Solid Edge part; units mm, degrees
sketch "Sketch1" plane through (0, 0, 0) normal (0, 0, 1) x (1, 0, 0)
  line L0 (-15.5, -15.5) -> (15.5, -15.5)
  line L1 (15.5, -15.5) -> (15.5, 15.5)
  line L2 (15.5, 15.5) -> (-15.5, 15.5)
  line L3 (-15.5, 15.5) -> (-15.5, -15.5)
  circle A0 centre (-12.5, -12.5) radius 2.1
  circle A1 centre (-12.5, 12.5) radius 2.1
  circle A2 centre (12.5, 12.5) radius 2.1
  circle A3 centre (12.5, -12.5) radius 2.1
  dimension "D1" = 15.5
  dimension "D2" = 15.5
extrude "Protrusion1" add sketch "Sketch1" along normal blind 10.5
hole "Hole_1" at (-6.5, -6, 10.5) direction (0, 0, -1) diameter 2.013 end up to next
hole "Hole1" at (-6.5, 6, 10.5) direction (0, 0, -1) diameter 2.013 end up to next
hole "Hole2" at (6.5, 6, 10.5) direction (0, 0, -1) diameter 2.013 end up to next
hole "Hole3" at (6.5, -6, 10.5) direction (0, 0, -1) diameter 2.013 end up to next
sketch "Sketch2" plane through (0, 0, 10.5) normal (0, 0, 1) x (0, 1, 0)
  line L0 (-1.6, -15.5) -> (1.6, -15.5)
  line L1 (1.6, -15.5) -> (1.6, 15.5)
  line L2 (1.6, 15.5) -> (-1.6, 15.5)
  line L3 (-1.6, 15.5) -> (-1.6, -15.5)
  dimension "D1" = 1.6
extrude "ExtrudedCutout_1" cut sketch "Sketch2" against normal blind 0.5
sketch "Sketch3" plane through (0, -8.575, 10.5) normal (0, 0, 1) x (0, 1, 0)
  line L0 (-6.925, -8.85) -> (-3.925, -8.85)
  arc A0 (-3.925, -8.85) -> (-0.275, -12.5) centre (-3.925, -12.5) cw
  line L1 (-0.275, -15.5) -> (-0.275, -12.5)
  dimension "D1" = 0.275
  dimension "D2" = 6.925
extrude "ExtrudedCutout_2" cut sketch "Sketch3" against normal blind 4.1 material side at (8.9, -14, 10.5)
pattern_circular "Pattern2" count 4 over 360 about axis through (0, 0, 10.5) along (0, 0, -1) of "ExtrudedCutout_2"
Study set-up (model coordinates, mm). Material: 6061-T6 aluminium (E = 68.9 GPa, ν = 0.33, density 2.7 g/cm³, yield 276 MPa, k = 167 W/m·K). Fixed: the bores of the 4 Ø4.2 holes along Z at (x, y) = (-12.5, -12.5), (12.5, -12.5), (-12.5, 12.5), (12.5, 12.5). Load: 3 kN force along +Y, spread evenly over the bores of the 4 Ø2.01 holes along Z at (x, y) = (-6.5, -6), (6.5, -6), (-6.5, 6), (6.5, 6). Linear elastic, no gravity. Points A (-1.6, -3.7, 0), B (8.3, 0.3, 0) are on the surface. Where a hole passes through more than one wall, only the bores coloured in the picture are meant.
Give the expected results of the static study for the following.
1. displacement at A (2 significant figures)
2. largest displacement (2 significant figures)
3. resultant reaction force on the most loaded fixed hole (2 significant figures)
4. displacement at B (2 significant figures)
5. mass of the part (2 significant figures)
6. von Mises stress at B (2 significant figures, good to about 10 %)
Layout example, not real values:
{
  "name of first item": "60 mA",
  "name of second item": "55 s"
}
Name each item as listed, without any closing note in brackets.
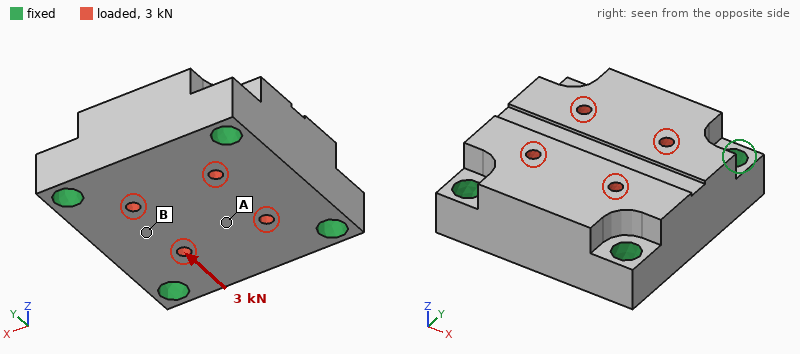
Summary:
{
  "displacement at A": "1.8 µm",
  "largest displacement": "2.3 µm",
  "resultant reaction force on the most loaded fixed hole": "810 N",
  "displacement at B": "1.4 µm",
  "mass of the part": "24 g",
  "von Mises stress at B": "7.9 MPa"
}
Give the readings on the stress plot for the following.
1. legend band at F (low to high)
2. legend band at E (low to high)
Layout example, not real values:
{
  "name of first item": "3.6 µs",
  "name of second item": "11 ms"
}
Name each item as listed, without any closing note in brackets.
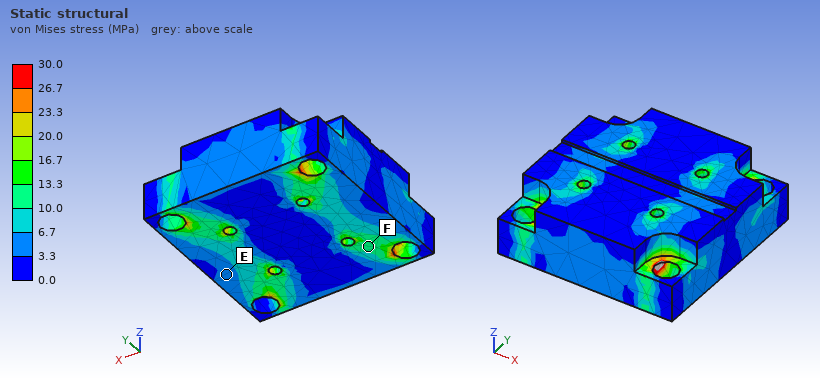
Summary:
{
  "legend band at F": "10.0 to 13.3 MPa",
  "legend band at E": "3.3 to 6.7 MPa"
}
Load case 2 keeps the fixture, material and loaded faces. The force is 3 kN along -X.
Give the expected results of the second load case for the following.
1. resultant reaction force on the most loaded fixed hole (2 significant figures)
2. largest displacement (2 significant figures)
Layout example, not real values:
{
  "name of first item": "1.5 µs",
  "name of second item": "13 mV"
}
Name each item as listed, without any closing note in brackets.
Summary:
{
  "resultant reaction force on the most loaded fixed hole": "810 N",
  "largest displacement": "2.4 µm"
}
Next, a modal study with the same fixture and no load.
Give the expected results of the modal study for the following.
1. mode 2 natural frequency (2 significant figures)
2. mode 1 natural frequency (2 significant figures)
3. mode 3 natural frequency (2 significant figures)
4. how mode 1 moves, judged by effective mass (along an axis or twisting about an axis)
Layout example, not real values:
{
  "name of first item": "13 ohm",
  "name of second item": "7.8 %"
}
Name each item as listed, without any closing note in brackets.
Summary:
{
  "mode 2 natural frequency": "45 kHz",
  "mode 1 natural frequency": "33 kHz",
  "mode 3 natural frequency": "45 kHz",
  "how mode 1 moves, judged by effective mass": "along Z"
}
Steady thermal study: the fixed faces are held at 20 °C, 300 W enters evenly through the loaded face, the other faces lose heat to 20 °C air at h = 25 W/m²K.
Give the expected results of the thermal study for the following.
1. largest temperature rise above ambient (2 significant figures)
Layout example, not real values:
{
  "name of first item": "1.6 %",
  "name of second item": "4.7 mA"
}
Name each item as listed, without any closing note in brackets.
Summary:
{
  "largest temperature rise above ambient": "45 K"
}
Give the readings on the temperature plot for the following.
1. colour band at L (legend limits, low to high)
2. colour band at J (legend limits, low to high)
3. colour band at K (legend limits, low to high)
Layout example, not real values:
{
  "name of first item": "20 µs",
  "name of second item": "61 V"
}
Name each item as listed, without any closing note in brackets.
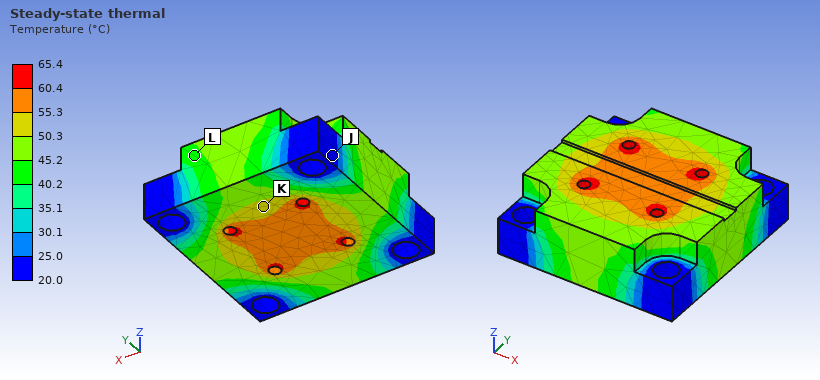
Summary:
{
  "colour band at L": "40.2 to 45.2 °C",
  "colour band at J": "20.0 to 25.0 °C",
  "colour band at K": "50.3 to 55.3 °C"
}
